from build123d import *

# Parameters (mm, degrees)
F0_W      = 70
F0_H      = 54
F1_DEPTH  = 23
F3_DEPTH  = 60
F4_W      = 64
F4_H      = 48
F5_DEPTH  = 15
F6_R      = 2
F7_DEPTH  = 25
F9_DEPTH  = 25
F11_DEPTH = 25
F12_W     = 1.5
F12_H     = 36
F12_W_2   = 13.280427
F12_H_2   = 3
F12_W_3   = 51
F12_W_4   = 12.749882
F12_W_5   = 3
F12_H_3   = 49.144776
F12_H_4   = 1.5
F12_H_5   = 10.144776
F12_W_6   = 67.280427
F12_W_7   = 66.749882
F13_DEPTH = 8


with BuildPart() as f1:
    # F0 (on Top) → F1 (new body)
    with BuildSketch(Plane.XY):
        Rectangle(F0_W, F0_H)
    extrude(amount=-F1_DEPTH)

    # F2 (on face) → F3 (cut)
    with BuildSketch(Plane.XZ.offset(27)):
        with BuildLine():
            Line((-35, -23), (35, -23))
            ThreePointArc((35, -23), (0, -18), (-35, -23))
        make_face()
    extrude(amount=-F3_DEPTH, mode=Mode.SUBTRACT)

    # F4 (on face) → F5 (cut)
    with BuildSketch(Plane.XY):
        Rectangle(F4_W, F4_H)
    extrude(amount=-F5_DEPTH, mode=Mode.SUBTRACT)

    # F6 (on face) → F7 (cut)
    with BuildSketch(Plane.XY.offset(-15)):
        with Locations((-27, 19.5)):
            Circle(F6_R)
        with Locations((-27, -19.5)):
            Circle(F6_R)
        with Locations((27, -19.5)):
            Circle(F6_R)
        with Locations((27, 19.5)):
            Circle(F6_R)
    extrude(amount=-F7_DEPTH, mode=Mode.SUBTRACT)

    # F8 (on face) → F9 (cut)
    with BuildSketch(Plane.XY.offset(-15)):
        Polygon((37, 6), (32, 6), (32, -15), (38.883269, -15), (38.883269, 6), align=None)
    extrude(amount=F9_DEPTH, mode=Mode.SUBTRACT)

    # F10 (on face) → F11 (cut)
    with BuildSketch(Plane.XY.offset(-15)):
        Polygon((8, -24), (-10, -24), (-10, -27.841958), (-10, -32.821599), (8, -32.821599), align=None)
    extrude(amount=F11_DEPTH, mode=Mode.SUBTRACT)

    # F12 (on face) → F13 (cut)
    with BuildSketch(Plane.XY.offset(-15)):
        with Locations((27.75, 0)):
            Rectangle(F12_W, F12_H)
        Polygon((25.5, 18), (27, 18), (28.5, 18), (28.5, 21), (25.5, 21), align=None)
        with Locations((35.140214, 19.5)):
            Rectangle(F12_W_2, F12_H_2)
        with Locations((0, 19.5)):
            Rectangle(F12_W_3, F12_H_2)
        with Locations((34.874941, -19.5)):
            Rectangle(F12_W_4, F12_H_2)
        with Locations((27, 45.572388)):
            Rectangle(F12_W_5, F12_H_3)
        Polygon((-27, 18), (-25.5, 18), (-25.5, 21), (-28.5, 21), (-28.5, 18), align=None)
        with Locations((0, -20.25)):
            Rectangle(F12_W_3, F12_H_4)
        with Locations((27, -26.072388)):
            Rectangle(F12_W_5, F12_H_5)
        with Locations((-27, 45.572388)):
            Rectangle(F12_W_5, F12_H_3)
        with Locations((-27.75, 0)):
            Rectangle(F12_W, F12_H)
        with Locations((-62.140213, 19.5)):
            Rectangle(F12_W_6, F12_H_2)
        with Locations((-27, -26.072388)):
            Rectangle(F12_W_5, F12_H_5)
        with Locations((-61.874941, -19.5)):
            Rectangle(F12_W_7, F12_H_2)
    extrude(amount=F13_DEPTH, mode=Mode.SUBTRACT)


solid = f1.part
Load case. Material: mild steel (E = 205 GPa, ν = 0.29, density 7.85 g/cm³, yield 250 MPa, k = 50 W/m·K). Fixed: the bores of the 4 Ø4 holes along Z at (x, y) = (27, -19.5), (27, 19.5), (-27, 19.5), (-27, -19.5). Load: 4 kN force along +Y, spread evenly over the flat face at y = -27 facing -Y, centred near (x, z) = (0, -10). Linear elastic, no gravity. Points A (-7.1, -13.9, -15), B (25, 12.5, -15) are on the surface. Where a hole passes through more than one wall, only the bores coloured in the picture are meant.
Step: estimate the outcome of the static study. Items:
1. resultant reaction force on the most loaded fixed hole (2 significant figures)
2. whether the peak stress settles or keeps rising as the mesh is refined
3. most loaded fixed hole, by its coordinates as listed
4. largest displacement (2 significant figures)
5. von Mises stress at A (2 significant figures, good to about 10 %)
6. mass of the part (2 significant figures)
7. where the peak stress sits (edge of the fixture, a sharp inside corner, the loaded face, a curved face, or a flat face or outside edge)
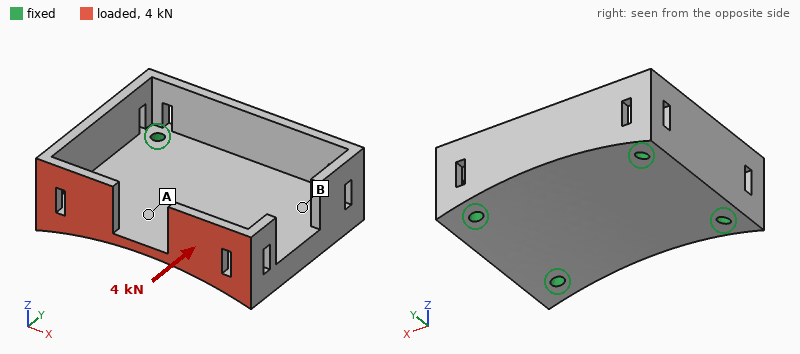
1.6 kN
keeps rising
(27, -19.5)
84 µm
27 MPa
200 g
edge of the fixture
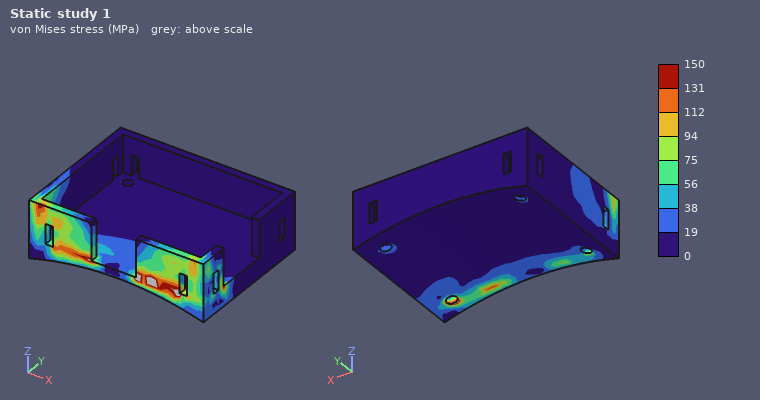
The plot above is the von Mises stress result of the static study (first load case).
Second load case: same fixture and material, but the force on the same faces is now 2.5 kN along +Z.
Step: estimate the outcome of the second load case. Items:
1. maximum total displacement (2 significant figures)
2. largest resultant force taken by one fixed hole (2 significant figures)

31 µm
1.4 kN
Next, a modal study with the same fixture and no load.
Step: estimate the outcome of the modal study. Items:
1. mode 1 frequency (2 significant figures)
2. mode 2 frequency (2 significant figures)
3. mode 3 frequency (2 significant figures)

7600 Hz
8500 Hz
9100 Hz
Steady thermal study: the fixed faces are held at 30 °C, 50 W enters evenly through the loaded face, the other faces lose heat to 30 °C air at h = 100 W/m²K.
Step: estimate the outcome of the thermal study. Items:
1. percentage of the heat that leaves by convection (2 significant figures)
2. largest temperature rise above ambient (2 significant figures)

26 %
60 K
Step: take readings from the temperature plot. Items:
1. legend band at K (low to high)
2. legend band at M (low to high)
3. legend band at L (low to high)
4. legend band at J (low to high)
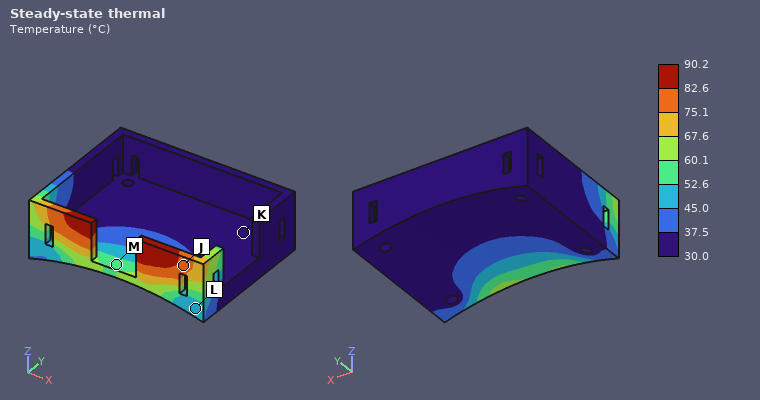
30.0 to 37.5 °C
52.6 to 60.1 °C
45.0 to 52.6 °C
75.1 to 82.6 °C
